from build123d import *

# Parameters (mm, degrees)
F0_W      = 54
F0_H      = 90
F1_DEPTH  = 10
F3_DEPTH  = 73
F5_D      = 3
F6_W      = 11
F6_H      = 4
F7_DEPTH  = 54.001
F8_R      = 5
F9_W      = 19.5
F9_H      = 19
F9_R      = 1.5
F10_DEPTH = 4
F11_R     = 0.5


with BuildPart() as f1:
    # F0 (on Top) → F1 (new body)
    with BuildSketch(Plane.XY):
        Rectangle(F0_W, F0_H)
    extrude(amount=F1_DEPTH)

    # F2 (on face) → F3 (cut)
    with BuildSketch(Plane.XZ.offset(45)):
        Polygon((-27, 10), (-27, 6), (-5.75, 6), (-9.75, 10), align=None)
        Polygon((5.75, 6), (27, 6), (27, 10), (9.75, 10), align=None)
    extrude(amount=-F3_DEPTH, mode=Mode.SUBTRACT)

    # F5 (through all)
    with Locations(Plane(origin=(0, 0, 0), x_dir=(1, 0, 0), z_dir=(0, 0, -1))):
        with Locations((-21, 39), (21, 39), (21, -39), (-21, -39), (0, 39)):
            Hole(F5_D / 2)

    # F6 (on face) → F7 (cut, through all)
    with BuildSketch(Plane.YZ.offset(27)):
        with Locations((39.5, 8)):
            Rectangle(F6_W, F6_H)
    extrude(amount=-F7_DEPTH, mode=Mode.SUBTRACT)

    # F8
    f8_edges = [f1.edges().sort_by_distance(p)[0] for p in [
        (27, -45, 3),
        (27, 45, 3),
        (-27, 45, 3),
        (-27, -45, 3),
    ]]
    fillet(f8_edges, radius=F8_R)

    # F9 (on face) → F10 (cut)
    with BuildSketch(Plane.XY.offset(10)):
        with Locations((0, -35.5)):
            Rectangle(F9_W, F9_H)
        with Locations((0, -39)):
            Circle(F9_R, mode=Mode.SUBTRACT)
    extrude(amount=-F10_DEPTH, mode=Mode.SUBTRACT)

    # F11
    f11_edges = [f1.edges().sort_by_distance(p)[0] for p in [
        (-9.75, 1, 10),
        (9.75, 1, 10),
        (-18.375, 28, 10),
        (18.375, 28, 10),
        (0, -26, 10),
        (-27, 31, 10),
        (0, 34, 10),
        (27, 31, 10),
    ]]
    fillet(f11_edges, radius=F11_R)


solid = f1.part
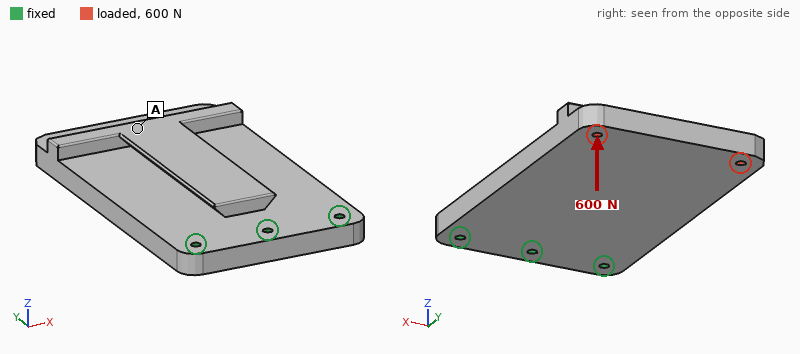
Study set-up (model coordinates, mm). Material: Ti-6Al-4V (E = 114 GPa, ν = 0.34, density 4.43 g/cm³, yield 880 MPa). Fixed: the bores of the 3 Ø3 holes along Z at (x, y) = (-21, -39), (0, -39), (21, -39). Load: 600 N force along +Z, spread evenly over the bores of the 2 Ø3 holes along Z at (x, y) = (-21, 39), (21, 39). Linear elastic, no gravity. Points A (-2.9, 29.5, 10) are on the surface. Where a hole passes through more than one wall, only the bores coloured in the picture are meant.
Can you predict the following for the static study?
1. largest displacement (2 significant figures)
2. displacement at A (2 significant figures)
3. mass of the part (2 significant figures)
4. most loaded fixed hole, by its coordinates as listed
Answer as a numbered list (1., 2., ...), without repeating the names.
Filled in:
1. 0.75 mm
2. 0.57 mm
3. 150 g
4. (0, -39)
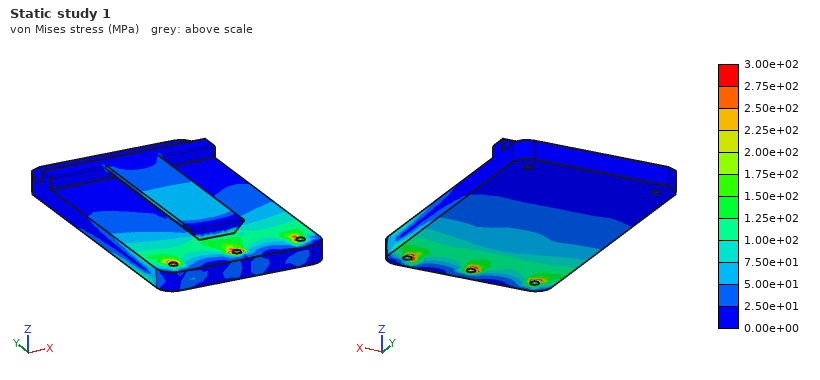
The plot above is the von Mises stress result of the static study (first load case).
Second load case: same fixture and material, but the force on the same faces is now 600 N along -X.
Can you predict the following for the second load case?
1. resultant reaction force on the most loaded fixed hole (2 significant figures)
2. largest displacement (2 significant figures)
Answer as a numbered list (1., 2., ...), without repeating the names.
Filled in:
1. 1.1 kN
2. 18 µm
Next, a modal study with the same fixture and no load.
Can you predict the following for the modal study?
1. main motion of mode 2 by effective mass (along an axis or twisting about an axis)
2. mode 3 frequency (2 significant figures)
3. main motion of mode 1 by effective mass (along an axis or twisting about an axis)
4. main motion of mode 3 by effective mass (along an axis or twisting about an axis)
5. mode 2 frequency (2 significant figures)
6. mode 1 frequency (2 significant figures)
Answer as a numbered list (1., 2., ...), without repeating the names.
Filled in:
1. twisting about Y
2. 4400 Hz
3. along Z
4. along X
5. 2600 Hz
6. 700 Hz
